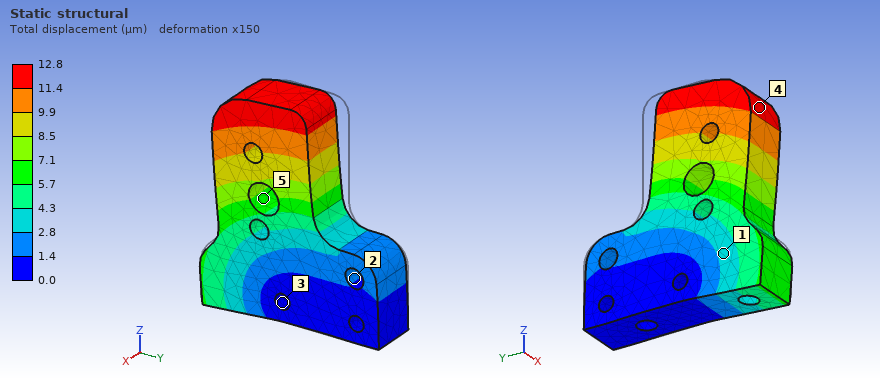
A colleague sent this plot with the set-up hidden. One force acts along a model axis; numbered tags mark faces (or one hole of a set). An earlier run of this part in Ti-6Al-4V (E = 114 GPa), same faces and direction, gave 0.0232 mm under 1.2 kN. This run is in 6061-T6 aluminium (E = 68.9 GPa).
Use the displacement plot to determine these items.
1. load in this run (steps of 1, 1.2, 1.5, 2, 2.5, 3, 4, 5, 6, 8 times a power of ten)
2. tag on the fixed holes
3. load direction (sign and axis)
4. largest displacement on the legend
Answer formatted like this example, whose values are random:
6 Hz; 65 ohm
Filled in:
400 N; 3; -Y; 12.8 µm
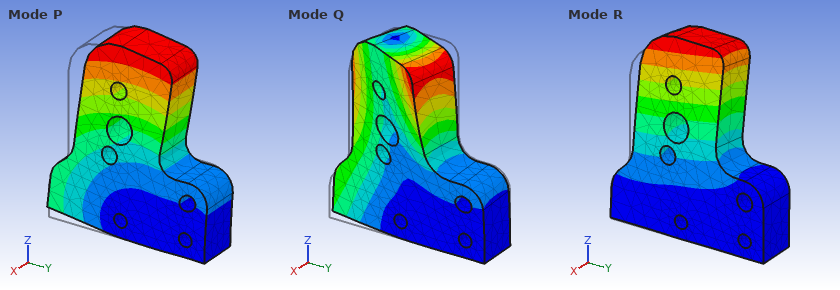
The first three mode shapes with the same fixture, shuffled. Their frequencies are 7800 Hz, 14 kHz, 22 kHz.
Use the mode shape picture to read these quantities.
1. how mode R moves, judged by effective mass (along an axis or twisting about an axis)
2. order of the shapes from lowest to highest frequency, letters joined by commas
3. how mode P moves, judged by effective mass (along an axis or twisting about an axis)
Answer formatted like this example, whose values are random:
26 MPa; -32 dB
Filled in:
along X; R, P, Q; along Y
